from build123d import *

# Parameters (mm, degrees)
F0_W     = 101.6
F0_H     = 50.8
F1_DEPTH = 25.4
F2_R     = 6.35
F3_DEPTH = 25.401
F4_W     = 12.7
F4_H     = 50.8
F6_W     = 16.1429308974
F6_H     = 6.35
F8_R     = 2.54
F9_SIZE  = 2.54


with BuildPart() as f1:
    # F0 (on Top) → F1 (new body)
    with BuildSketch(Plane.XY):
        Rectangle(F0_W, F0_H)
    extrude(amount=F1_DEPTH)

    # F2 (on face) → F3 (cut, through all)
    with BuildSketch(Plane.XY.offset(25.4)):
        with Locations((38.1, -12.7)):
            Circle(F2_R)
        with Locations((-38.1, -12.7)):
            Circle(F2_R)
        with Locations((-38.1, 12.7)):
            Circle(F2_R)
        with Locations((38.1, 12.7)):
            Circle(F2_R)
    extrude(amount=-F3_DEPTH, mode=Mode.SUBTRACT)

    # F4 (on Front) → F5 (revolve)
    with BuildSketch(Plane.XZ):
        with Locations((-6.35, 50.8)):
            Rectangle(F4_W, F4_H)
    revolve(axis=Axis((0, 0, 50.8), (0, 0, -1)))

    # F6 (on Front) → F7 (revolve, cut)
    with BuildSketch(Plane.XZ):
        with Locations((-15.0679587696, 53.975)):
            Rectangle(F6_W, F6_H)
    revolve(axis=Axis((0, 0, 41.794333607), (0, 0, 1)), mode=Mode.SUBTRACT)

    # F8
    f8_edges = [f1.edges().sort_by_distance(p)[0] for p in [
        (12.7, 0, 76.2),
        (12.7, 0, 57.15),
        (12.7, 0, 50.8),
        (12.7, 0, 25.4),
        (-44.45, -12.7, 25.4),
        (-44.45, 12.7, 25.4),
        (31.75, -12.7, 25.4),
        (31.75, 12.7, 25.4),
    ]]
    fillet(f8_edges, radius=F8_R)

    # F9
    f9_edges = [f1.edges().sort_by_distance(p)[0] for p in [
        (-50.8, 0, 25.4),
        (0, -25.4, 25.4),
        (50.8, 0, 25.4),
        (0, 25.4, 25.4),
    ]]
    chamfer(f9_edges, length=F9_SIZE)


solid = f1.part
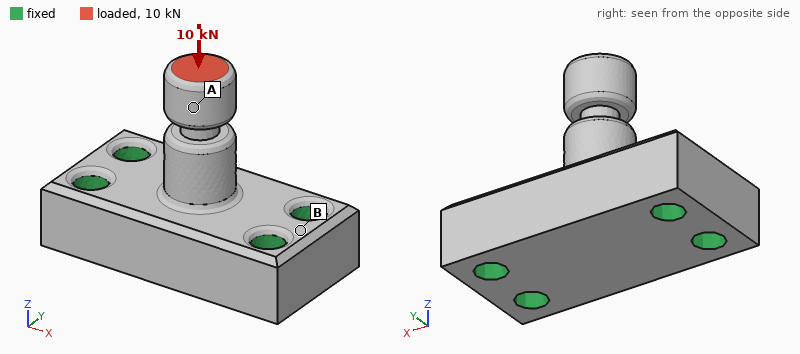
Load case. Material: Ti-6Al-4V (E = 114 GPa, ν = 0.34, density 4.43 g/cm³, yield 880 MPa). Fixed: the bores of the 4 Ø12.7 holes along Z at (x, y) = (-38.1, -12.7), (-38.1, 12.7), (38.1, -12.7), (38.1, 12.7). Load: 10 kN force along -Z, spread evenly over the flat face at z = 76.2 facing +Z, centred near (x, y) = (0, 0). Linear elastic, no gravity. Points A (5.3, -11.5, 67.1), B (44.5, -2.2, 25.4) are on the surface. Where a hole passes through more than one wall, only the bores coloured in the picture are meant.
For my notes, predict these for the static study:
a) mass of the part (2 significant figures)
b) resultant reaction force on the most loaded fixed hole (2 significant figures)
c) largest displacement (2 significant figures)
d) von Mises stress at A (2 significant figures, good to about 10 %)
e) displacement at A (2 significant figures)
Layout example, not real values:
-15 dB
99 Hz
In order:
620 g
2.6 kN
20 µm
13 MPa
18 µm
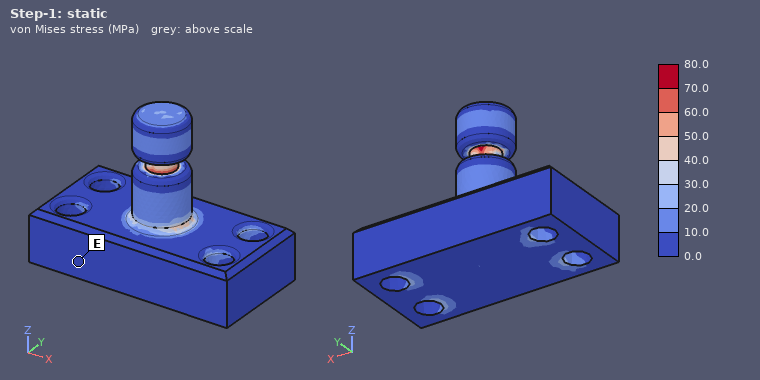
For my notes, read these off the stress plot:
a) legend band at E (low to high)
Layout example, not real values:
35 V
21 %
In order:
0.0 to 10.0 MPa
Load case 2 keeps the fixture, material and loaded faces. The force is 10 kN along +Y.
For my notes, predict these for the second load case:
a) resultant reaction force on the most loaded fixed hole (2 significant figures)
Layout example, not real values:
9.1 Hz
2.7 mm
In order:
8.6 kN
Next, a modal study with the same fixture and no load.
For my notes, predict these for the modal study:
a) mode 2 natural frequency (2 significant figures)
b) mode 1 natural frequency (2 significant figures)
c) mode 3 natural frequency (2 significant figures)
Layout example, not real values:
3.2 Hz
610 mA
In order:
4500 Hz
4200 Hz
9700 Hz
